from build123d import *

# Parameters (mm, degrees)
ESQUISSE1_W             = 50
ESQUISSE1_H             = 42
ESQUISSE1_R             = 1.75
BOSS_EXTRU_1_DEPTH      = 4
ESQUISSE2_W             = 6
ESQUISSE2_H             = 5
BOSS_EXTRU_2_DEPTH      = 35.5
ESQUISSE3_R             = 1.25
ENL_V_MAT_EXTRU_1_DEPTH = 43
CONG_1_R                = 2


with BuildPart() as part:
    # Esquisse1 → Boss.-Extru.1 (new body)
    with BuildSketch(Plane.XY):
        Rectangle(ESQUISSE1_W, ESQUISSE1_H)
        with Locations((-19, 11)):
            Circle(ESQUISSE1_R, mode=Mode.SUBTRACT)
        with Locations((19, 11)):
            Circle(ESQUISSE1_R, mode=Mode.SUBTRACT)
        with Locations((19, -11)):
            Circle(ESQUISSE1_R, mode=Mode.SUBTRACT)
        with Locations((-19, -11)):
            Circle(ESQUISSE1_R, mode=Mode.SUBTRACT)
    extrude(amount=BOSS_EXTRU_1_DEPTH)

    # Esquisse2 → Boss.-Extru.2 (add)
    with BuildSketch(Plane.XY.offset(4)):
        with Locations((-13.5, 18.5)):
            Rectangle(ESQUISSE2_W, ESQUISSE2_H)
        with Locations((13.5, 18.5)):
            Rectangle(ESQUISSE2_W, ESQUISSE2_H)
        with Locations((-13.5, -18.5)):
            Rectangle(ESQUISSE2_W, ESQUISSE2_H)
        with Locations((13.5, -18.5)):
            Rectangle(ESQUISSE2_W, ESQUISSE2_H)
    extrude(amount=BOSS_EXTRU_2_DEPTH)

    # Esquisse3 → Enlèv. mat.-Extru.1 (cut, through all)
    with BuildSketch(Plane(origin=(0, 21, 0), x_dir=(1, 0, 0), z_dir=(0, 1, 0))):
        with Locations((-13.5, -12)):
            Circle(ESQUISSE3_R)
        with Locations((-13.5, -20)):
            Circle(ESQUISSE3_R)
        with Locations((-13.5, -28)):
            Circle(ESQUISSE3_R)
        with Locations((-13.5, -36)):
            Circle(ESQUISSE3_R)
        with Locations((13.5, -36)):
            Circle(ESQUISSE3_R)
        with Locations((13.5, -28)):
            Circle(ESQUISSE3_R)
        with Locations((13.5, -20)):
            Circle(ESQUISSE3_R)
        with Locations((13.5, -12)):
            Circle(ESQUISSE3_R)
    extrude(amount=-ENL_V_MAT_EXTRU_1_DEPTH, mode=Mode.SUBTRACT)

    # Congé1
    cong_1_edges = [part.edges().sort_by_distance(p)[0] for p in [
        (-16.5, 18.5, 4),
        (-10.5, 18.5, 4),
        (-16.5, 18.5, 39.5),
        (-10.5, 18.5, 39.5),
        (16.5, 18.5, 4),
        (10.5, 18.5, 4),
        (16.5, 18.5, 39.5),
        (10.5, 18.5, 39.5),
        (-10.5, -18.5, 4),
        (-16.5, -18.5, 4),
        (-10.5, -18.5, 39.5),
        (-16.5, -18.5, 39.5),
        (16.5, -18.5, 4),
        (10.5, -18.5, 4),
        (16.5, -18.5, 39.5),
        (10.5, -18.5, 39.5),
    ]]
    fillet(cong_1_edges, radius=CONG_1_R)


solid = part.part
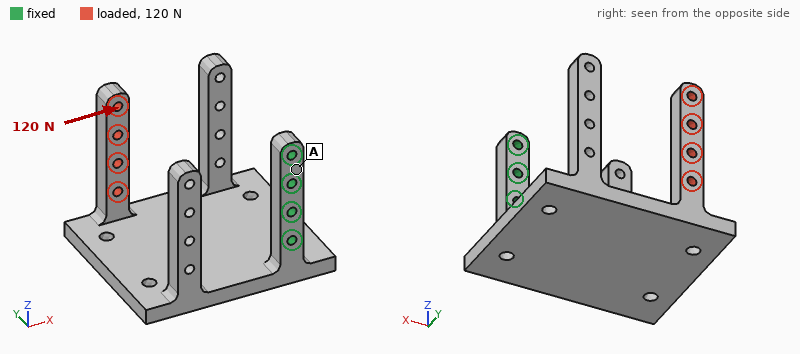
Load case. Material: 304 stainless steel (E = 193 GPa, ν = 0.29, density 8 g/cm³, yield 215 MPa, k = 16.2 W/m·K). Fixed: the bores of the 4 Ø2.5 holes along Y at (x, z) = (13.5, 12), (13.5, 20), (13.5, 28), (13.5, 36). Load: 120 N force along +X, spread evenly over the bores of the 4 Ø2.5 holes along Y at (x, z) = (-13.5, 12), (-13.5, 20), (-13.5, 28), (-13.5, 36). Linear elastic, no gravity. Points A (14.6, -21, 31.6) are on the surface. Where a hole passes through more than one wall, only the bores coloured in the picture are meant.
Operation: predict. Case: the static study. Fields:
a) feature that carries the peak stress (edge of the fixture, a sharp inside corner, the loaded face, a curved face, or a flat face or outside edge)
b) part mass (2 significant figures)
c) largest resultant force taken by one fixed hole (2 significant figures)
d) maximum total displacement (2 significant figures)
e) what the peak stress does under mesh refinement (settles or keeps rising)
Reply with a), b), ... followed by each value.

a) edge of the fixture
b) 97 g
c) 61 N
d) 0.38 mm
e) keeps rising
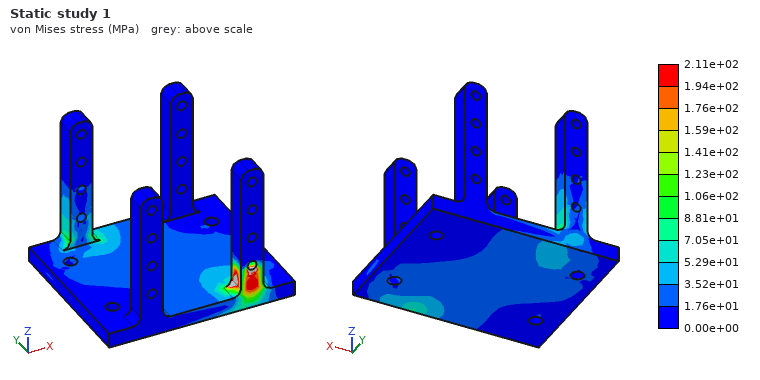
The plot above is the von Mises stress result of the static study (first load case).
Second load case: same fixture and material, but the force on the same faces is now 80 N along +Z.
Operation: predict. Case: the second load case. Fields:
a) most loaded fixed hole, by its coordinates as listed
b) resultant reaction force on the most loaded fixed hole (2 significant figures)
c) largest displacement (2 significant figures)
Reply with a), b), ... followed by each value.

a) (13.5, 12)
b) 120 N
c) 0.28 mm
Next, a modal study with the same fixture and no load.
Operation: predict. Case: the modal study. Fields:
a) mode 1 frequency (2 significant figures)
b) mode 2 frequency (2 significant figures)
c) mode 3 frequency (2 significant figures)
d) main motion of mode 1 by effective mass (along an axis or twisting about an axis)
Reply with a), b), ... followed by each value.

a) 540 Hz
b) 560 Hz
c) 900 Hz
d) along Z
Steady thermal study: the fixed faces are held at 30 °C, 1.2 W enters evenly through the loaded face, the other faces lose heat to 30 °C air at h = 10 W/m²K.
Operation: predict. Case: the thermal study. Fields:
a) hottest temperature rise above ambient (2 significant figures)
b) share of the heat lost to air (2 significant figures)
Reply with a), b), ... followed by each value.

a) 61 K
b) 77 %
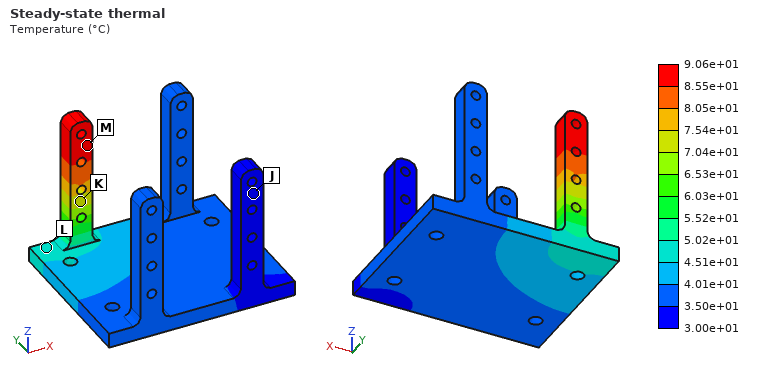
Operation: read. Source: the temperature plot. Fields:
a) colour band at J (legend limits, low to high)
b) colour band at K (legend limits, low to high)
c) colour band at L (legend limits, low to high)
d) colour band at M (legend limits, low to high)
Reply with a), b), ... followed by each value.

a) 3.00e+01 to 3.50e+01 °C
b) 7.04e+01 to 7.54e+01 °C
c) 4.51e+01 to 5.02e+01 °C
d) 8.55e+01 to 9.06e+01 °C
